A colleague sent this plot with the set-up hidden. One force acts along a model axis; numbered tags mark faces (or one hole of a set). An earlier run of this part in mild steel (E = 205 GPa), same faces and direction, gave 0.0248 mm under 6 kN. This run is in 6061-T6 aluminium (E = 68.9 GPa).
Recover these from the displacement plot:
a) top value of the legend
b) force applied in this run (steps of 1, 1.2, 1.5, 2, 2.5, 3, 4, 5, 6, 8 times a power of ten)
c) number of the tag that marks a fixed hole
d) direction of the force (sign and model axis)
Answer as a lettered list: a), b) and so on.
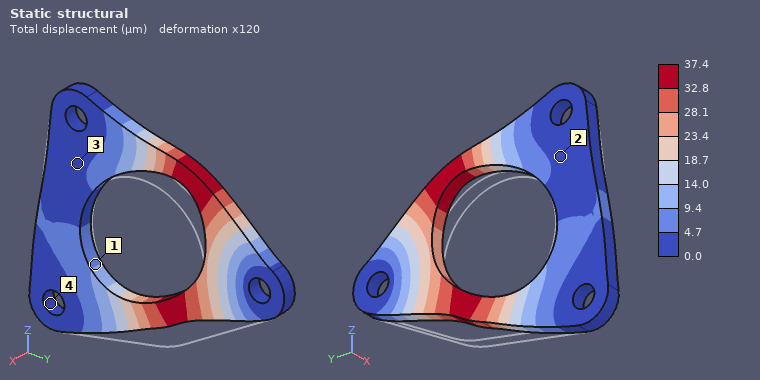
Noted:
a) 37.4 µm
b) 3 kN
c) 4
d) +Z
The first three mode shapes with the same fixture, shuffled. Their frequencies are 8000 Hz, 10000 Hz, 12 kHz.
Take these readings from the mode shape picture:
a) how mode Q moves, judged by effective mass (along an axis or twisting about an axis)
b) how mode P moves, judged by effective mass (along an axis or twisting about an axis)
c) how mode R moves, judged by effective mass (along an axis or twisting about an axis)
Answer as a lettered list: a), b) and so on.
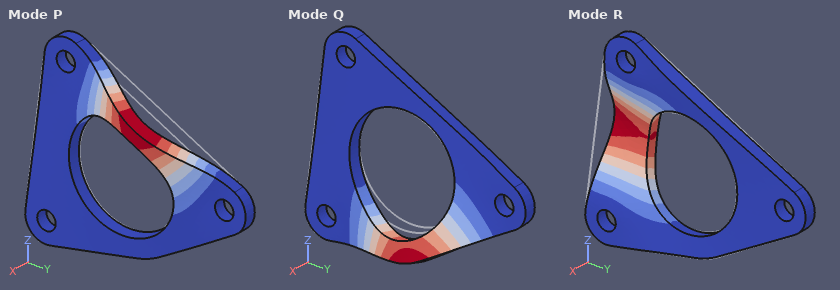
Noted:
a) along X
b) along X
c) along X
